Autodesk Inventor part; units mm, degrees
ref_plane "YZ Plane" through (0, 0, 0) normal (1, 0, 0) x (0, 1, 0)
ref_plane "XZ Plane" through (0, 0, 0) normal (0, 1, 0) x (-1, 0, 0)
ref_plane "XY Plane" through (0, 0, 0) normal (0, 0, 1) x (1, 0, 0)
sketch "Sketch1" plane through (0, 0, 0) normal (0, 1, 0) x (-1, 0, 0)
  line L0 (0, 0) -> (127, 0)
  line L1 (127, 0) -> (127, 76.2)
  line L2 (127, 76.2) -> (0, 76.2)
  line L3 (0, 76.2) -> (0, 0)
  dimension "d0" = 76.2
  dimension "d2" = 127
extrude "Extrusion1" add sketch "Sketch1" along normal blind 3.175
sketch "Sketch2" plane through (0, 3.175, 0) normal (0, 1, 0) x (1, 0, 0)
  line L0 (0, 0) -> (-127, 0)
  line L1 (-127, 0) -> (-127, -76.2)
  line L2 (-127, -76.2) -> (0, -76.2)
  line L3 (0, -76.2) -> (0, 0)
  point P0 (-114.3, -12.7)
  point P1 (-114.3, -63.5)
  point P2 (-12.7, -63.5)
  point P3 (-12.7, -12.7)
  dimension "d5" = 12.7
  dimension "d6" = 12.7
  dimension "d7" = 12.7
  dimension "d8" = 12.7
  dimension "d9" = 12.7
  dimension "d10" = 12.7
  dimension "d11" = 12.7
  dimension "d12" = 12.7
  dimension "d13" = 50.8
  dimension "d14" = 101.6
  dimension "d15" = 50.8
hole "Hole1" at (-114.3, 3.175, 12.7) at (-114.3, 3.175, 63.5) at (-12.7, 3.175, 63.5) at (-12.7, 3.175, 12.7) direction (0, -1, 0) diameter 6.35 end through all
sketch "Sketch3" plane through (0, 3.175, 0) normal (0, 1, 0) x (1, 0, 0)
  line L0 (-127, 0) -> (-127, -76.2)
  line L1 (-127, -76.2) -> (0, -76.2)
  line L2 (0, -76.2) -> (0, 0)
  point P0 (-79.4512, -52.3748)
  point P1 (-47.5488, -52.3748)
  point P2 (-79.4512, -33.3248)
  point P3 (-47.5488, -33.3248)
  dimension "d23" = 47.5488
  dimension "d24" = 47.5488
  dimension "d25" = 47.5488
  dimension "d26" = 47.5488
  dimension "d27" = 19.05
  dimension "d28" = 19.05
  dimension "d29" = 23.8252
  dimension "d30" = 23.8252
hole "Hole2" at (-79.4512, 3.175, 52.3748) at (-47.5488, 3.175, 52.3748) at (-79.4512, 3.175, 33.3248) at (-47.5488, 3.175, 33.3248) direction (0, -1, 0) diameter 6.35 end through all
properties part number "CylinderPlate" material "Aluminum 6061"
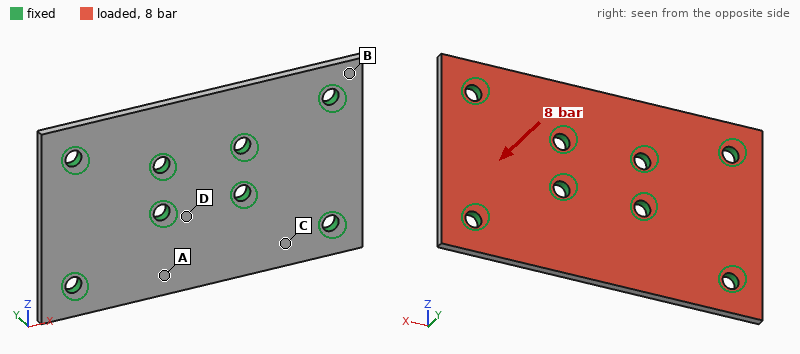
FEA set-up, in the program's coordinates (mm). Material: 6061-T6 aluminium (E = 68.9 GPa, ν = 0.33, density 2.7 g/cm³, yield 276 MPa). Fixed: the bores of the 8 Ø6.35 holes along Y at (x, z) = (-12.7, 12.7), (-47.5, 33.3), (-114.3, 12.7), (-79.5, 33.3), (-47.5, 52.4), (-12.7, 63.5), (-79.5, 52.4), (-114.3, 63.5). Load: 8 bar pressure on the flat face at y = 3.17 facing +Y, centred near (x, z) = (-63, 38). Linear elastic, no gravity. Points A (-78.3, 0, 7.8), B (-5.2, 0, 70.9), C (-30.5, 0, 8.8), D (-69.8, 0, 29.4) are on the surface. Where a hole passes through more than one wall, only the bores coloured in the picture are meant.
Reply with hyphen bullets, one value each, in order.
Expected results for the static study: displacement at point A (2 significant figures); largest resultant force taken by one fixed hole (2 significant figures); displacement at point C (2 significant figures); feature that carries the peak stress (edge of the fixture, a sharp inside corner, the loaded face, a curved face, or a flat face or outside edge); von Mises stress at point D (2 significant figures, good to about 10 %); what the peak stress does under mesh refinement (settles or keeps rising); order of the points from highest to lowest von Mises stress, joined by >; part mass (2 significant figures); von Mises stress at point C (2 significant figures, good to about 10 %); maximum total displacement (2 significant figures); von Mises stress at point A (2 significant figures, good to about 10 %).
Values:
- 0.22 mm
- 1.1 kN
- 0.098 mm
- edge of the fixture
- 79 MPa
- keeps rising
- D > C > A > B
- 81 g
- 53 MPa
- 0.36 mm
- 40 MPa
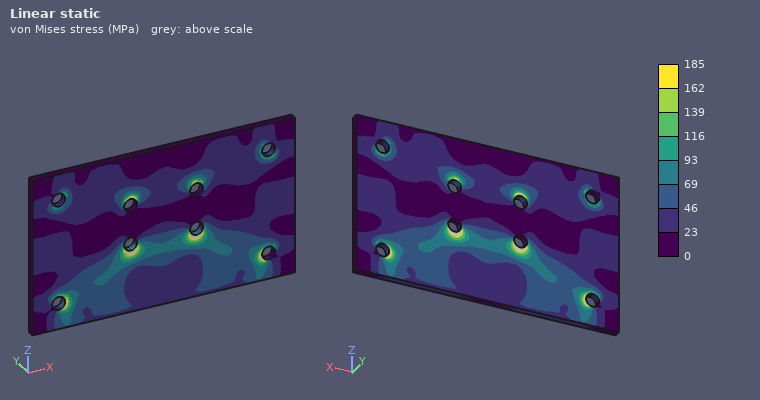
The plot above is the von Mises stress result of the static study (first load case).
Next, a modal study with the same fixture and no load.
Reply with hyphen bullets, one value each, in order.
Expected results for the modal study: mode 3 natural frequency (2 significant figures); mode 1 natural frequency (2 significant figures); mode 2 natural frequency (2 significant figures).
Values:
- 6100 Hz
- 3500 Hz
- 5600 Hz
